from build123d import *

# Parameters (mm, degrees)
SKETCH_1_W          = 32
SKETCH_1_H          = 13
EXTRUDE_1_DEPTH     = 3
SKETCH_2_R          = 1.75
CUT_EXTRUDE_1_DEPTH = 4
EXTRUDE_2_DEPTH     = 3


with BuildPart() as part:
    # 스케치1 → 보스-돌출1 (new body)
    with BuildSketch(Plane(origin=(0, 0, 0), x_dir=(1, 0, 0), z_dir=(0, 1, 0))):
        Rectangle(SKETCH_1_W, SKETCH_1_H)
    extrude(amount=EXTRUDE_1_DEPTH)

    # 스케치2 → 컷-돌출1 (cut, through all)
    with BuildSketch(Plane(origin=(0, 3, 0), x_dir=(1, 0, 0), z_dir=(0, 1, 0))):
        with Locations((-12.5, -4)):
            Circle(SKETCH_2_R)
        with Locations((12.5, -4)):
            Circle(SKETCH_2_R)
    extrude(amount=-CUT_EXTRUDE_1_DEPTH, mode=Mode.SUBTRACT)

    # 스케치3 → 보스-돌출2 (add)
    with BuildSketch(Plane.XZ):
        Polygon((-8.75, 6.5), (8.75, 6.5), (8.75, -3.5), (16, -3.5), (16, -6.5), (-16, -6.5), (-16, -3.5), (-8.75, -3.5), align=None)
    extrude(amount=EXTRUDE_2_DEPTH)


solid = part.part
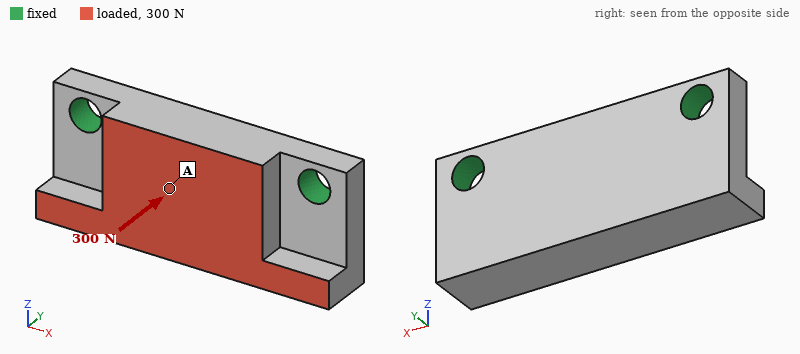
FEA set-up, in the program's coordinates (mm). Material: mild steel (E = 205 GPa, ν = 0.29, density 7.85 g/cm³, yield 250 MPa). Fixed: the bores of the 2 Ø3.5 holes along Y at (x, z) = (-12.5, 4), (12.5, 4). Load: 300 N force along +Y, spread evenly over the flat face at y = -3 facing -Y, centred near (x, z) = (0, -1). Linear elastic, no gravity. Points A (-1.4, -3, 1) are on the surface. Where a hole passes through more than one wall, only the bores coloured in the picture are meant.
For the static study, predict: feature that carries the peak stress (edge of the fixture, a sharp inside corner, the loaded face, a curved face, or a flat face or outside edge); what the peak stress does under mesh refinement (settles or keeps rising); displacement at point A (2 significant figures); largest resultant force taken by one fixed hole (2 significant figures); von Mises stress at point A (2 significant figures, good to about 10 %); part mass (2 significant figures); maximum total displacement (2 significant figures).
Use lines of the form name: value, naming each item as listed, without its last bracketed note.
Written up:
feature that carries the peak stress: edge of the fixture
what the peak stress does under mesh refinement: keeps rising
displacement at point A: 2.1 µm
largest resultant force taken by one fixed hole: 160 N
von Mises stress at point A: 8.2 MPa
part mass: 16 g
maximum total displacement: 4.3 µm
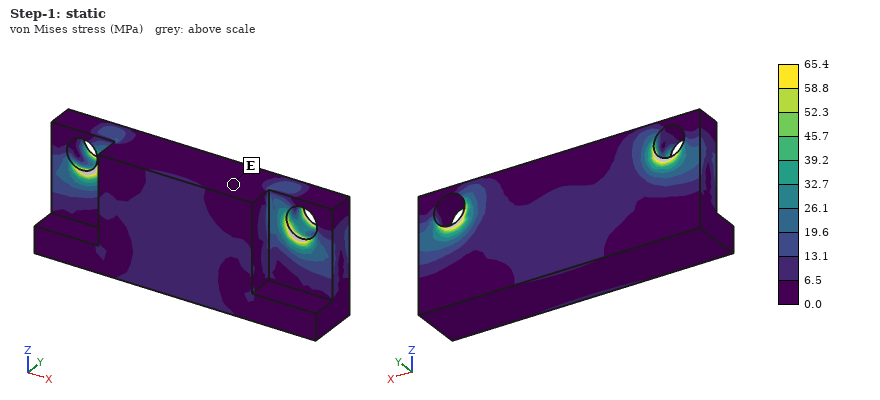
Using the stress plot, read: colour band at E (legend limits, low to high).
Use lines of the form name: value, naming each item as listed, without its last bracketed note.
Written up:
colour band at E: 0.0 to 6.5 MPa
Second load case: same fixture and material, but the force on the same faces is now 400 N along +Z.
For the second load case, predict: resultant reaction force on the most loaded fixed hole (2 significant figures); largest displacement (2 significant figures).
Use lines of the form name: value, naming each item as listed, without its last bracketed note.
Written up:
resultant reaction force on the most loaded fixed hole: 220 N
largest displacement: 6.2 µm
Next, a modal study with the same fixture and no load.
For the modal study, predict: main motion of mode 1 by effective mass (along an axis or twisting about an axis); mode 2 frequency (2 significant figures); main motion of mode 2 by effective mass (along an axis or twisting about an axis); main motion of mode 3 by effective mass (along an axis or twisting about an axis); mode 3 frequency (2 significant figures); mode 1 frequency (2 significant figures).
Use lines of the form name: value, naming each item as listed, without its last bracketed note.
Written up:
main motion of mode 1 by effective mass: along Y
mode 2 frequency: 30 kHz
main motion of mode 2 by effective mass: twisting about Z
main motion of mode 3 by effective mass: along Y
mode 3 frequency: 33 kHz
mode 1 frequency: 13 kHz
